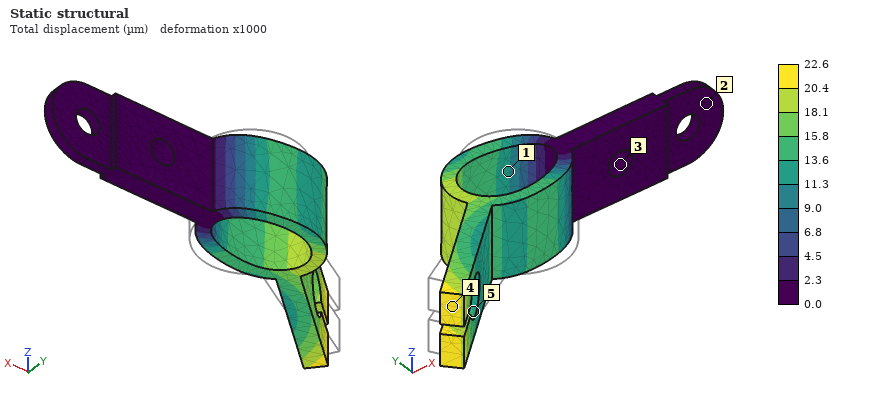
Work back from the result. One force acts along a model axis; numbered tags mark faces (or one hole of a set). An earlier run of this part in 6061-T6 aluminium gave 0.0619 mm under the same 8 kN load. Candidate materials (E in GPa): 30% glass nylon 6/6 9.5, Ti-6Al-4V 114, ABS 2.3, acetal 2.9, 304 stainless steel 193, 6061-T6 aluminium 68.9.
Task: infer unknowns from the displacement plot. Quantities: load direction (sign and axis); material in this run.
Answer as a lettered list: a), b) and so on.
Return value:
a) -X
b) 304 stainless steel
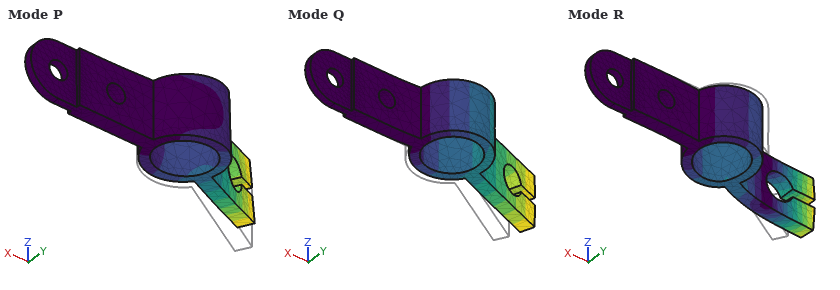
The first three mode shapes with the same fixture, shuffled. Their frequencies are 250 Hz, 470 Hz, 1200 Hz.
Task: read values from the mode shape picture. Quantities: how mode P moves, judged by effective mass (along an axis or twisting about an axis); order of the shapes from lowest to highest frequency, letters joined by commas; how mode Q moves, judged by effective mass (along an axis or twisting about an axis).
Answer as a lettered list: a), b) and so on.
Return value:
a) along Z
b) Q, P, R
c) along Y
